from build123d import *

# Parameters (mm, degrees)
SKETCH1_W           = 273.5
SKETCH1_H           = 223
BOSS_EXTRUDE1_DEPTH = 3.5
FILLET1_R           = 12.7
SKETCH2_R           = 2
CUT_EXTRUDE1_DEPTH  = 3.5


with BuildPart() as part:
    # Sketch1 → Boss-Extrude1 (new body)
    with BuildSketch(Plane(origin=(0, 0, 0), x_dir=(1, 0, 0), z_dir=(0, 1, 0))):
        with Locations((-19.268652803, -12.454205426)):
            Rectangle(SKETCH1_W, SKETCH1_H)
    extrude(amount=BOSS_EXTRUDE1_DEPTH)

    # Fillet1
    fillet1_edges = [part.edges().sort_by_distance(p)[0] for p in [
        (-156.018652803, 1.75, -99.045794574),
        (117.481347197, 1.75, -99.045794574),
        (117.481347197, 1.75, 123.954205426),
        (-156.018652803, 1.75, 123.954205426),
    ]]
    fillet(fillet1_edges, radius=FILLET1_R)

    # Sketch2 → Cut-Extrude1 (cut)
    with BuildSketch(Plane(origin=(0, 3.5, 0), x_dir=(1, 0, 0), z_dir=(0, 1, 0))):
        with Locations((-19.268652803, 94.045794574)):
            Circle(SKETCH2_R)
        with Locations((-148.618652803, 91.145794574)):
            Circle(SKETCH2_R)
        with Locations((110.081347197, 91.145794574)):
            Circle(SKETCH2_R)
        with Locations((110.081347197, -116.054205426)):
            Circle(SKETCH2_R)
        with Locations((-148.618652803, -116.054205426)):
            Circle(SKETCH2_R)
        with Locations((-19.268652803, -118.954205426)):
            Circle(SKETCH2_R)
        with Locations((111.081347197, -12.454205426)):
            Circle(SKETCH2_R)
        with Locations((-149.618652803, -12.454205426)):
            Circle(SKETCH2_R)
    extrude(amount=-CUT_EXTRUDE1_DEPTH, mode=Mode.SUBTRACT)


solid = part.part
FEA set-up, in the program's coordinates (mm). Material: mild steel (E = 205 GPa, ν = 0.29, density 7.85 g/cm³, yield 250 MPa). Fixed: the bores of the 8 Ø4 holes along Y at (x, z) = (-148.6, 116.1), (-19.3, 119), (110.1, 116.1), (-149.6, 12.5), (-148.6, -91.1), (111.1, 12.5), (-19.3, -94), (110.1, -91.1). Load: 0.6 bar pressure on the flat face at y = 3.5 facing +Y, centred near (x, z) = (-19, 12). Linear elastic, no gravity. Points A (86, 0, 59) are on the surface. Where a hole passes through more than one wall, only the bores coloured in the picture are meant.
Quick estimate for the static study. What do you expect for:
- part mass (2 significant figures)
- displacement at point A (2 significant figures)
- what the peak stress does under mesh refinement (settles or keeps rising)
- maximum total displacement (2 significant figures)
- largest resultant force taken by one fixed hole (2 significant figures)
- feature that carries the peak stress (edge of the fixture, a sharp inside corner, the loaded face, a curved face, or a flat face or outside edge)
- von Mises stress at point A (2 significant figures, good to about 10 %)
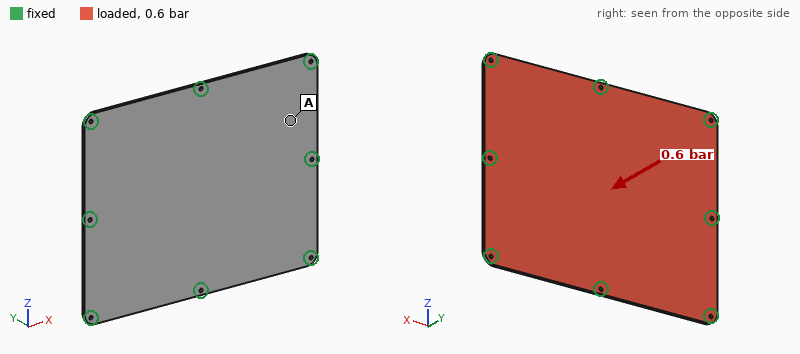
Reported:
1.7 kg
0.13 mm
keeps rising
0.47 mm
770 N
edge of the fixture
29 MPa
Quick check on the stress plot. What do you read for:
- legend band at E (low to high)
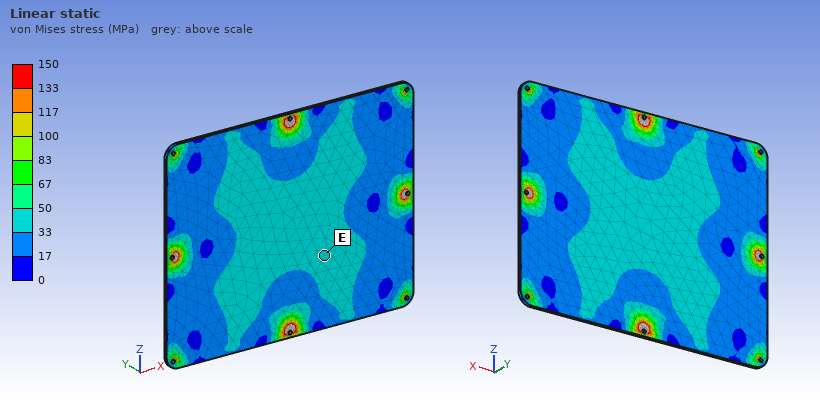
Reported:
33 to 50 MPa
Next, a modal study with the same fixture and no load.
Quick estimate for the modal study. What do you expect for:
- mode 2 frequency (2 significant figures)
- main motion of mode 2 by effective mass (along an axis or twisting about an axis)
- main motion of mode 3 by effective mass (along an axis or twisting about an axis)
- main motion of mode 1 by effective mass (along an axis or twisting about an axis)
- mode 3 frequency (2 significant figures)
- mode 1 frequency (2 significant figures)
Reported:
690 Hz
twisting about Z
twisting about X
along Y
850 Hz
430 Hz
